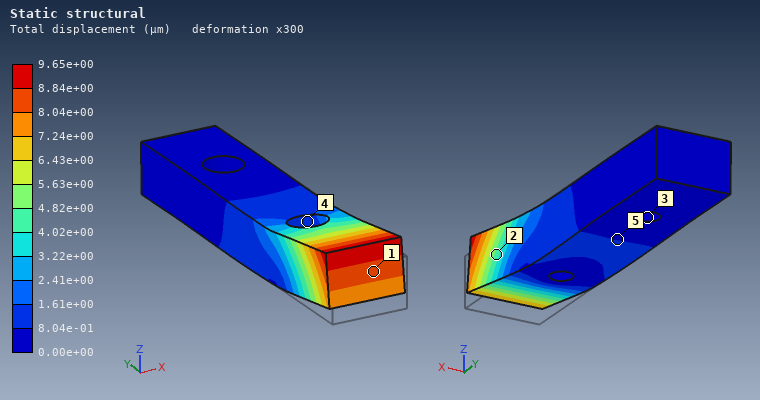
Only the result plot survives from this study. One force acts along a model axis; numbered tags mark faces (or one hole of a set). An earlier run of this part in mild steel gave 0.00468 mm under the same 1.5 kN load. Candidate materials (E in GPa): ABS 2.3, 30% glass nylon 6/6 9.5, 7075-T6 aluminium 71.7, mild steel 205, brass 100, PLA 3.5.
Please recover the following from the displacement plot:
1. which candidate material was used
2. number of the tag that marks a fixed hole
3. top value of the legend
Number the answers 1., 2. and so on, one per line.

1. brass
2. 3
3. 9.65e+00 µm
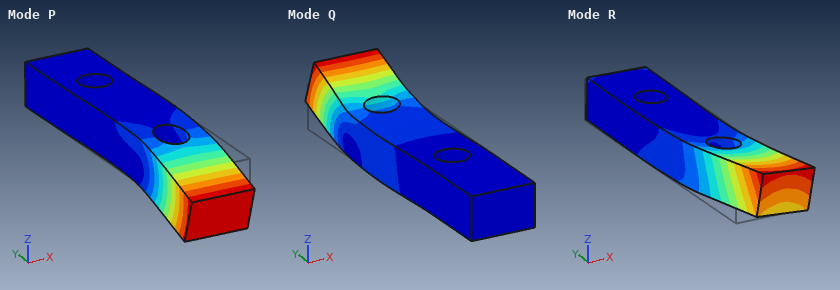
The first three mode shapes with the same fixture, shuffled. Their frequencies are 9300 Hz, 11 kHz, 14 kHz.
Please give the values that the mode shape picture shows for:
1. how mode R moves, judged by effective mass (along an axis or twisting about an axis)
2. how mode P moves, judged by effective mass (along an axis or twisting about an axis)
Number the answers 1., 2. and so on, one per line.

1. along X
2. along Z
